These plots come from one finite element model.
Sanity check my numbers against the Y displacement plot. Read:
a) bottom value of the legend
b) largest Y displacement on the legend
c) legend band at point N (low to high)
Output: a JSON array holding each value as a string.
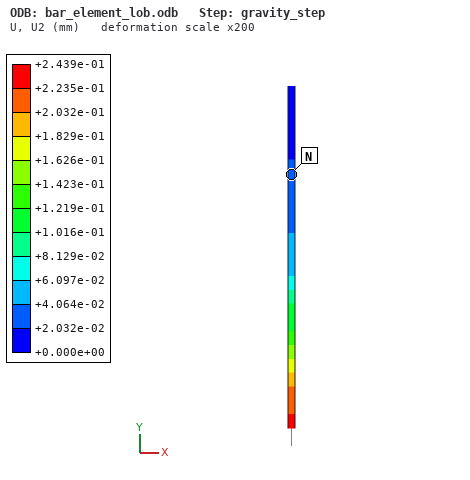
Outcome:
["+0.000e+00 mm", "+2.439e-01 mm", "+2.032e-02 to +4.064e-02 mm"]
